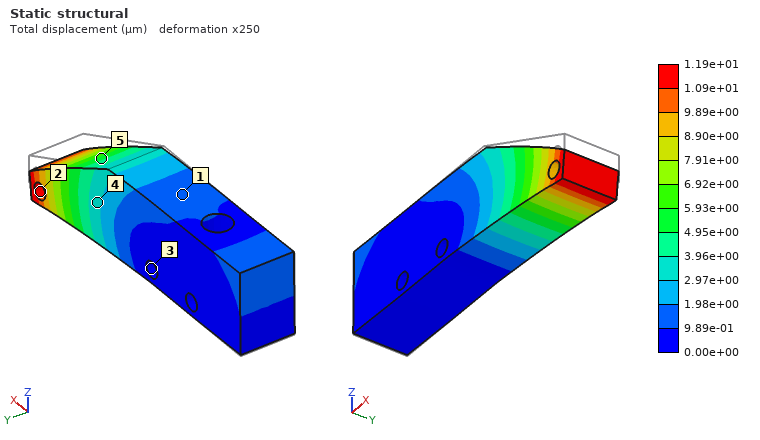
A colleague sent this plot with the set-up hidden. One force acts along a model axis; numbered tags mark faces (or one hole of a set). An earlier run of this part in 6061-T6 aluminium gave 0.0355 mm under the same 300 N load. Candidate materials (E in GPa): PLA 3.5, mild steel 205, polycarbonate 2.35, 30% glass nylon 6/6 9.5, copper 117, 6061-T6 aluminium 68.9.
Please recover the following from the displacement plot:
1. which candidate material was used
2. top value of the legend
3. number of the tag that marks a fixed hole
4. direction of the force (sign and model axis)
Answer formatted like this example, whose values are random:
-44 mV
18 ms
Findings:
mild steel
1.19e+01 µm
3
-Z
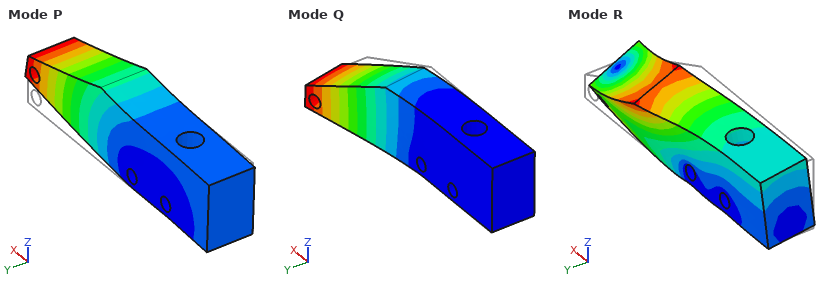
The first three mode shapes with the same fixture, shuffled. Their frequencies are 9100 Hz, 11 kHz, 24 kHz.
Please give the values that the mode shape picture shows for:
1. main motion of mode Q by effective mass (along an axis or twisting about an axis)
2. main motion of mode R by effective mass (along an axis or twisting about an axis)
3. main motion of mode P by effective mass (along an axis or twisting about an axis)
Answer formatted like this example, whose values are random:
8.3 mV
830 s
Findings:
along Y
along Y
along Z
